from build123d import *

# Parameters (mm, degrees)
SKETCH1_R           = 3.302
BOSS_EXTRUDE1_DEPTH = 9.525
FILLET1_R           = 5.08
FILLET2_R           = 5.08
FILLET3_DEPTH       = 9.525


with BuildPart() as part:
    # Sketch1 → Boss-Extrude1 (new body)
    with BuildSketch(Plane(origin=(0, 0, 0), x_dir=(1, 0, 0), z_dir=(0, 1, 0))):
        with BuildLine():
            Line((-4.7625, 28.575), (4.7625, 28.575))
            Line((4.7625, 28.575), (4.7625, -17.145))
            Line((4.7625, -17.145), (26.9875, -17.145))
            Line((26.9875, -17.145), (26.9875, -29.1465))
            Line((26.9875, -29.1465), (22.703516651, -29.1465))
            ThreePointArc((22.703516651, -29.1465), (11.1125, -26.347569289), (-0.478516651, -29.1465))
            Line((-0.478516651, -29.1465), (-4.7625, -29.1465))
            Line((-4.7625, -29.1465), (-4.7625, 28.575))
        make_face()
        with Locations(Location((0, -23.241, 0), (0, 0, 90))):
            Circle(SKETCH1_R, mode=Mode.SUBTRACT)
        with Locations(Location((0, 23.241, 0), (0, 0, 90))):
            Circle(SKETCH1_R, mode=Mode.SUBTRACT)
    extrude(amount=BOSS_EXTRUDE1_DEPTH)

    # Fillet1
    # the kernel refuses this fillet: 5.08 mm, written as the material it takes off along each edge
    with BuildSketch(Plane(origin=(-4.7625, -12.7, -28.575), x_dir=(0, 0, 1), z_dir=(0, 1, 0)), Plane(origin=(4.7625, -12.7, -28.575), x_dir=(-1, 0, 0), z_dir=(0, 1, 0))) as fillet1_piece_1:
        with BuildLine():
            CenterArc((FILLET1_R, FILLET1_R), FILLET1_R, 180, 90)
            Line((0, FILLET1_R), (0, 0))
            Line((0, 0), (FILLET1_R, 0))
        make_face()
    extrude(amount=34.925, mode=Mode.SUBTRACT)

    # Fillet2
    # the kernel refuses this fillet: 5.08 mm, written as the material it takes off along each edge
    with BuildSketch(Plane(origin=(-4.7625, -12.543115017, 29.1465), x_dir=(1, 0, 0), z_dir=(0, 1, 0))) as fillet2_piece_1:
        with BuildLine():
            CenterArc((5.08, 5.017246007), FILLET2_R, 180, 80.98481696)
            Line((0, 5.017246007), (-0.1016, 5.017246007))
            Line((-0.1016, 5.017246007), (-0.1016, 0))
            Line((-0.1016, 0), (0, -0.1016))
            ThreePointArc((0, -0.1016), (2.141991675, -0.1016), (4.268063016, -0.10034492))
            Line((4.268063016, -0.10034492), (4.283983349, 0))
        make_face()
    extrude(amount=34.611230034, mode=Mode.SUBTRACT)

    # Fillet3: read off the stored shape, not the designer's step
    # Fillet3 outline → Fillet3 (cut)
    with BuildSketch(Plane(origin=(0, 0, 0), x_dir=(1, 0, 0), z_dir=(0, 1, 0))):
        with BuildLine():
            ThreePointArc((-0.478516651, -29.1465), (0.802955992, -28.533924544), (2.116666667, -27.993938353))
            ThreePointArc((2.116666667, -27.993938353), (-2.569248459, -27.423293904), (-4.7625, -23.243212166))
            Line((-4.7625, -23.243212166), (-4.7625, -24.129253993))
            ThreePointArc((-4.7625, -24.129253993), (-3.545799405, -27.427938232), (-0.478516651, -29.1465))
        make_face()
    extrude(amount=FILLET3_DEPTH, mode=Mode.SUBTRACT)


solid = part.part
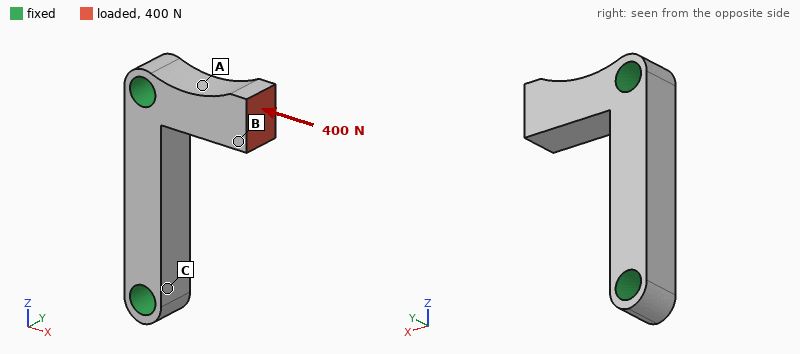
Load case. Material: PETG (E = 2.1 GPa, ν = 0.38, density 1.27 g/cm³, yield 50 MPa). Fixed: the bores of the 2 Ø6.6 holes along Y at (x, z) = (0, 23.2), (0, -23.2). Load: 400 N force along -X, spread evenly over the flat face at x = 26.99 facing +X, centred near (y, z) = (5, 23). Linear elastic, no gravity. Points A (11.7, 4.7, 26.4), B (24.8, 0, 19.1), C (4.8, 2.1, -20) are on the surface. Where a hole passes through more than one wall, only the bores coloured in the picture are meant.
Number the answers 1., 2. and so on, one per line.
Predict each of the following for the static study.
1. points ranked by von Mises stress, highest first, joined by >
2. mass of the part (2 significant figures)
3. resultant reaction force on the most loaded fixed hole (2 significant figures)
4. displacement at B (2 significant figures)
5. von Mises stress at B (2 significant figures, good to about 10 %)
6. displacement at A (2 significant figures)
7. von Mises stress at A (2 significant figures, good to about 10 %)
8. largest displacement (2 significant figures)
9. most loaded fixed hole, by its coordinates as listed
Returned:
1. A > B > C
2. 8.3 g
3. 400 N
4. 0.076 mm
5. 3.5 MPa
6. 0.034 mm
7. 9.6 MPa
8. 0.13 mm
9. (0, 23.2)
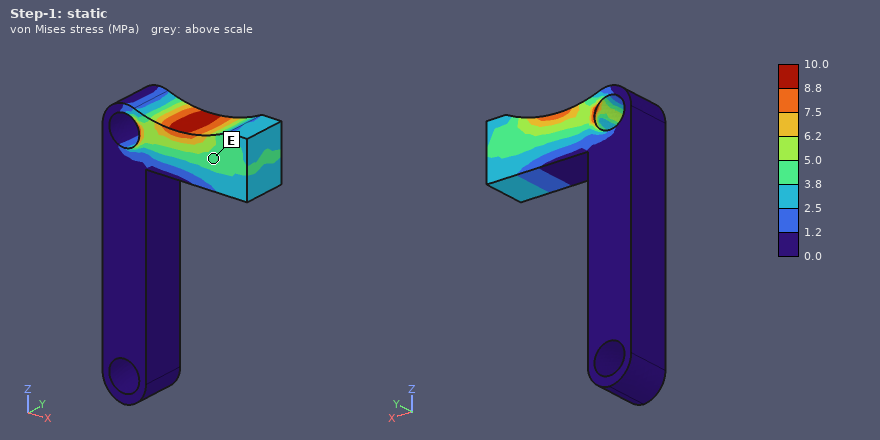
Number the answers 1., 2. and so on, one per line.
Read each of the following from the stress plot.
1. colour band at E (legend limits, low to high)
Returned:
1. 3.8 to 5.0 MPa
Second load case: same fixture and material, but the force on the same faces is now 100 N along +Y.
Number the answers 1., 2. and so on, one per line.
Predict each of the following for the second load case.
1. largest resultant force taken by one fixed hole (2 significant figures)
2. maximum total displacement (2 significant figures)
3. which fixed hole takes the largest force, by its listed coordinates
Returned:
1. 100 N
2. 0.39 mm
3. (0, 23.2)
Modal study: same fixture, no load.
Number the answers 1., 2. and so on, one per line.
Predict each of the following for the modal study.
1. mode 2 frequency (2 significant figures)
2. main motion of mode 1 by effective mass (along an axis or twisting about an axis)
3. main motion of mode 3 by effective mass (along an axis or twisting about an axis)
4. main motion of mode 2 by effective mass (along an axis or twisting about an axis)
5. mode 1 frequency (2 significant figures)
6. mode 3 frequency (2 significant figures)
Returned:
1. 2800 Hz
2. along Z
3. along X
4. along Y
5. 2600 Hz
6. 5400 Hz
